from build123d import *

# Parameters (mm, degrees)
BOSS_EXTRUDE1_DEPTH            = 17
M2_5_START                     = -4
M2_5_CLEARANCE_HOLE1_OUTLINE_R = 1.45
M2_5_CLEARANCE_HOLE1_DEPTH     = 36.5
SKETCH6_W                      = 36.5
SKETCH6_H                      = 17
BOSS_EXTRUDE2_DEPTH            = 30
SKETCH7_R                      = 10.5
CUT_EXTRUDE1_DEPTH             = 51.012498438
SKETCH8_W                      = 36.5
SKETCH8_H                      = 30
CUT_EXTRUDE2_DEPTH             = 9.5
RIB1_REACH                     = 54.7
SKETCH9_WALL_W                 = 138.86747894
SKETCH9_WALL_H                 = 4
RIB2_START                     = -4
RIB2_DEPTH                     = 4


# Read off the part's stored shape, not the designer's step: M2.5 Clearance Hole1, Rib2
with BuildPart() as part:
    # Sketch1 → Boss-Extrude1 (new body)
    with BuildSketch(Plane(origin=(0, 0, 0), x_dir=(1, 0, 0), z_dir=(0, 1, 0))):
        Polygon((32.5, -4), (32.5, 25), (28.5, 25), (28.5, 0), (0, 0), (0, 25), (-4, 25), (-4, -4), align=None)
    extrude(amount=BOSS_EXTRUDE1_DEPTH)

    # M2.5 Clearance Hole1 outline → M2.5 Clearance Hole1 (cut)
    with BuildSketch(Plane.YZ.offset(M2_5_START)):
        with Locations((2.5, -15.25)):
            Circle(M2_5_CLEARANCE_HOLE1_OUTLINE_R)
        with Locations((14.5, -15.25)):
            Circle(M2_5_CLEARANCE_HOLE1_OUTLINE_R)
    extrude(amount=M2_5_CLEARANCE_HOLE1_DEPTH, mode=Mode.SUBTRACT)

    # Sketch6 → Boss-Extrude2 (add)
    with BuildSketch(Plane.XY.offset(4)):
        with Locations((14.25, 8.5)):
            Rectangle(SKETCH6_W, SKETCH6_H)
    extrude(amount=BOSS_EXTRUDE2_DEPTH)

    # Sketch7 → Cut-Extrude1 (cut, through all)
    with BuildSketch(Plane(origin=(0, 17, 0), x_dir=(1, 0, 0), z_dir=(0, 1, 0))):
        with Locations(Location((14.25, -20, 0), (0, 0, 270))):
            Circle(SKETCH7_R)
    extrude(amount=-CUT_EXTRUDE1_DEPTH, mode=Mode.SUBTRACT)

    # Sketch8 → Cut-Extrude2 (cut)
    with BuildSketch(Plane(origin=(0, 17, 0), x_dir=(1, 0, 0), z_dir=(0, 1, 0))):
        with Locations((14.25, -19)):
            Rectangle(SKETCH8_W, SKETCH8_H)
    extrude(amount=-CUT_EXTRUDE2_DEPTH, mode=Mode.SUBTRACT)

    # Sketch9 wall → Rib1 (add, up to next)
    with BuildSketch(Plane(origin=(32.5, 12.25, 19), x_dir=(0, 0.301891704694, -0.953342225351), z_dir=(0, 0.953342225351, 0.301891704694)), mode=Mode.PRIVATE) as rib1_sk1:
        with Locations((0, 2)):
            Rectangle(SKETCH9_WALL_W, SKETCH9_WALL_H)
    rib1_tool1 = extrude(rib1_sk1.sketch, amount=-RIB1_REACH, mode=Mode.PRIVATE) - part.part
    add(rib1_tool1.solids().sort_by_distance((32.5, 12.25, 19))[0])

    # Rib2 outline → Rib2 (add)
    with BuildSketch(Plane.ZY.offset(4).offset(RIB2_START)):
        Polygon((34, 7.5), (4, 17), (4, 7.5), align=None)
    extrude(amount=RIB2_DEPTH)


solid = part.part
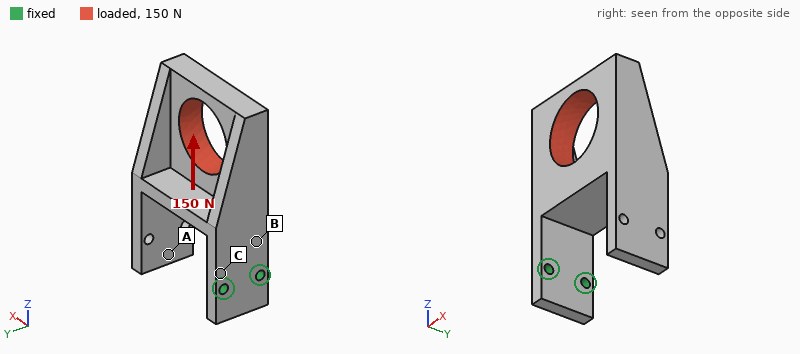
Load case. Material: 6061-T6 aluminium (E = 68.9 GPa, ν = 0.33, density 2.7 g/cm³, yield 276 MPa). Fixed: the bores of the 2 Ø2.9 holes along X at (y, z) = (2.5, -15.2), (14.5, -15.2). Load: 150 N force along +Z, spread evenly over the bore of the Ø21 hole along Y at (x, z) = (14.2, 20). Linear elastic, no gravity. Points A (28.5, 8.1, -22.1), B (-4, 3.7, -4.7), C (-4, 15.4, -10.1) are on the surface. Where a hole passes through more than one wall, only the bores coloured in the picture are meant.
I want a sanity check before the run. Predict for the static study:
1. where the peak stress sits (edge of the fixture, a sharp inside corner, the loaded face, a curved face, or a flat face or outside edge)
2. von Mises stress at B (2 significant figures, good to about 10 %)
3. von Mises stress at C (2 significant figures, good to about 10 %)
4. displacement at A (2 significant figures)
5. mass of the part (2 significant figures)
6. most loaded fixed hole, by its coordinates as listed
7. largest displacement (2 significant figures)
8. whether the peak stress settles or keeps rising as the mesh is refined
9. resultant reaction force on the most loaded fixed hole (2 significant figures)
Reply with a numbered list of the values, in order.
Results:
1. edge of the fixture
2. 48 MPa
3. 56 MPa
4. 0.23 mm
5. 34 g
6. (2.5, -15.2)
7. 0.36 mm
8. keeps rising
9. 130 N
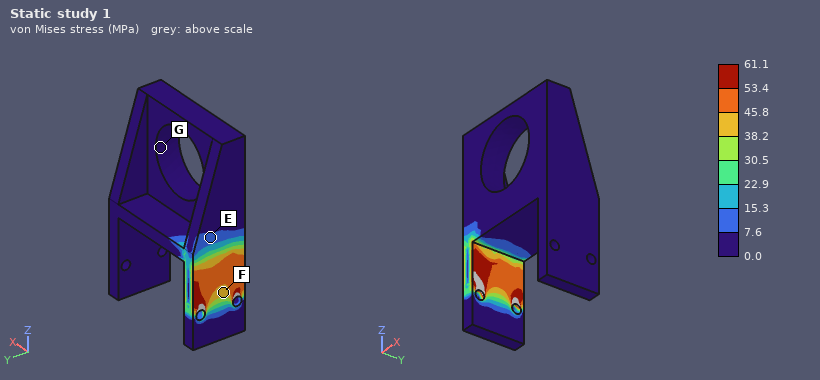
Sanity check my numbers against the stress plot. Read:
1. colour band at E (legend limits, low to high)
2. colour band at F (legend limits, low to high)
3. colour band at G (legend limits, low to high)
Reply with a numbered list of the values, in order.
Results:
1. 7.6 to 15.3 MPa
2. 38.2 to 45.8 MPa
3. 0.0 to 7.6 MPa
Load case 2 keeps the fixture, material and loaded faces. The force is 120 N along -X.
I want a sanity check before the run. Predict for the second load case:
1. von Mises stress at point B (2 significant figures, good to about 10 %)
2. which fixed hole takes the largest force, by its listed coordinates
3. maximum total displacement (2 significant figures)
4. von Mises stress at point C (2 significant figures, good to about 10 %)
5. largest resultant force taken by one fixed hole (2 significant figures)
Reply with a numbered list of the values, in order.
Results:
1. 64 MPa
2. (2.5, -15.2)
3. 0.48 mm
4. 79 MPa
5. 100 N
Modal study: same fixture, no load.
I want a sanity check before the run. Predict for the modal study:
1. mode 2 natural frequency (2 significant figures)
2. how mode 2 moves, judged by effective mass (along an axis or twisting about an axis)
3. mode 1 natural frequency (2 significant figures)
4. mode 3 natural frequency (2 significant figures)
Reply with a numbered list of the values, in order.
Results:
1. 1100 Hz
2. along Y
3. 570 Hz
4. 2800 Hz
